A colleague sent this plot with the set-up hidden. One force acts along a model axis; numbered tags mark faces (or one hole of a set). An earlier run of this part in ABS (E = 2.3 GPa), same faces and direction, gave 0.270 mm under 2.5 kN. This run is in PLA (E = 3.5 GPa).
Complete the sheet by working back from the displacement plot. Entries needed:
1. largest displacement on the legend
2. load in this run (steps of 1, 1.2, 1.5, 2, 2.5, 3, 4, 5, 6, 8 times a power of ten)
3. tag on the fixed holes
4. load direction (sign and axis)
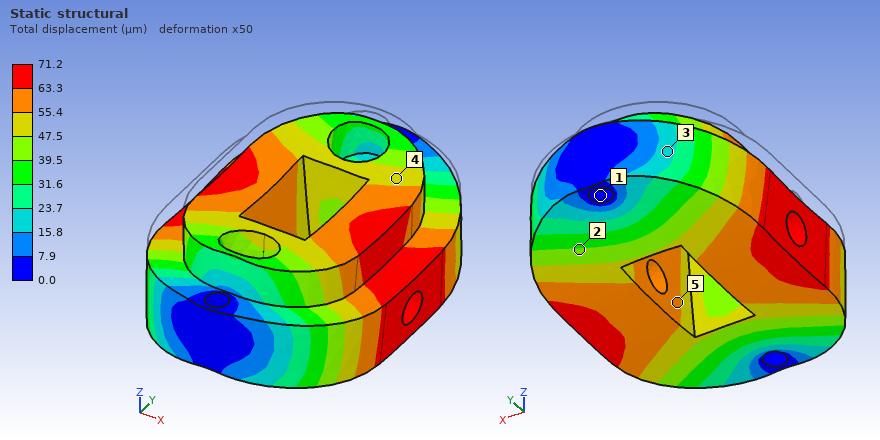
71.2 µm
1 kN
1
-Z
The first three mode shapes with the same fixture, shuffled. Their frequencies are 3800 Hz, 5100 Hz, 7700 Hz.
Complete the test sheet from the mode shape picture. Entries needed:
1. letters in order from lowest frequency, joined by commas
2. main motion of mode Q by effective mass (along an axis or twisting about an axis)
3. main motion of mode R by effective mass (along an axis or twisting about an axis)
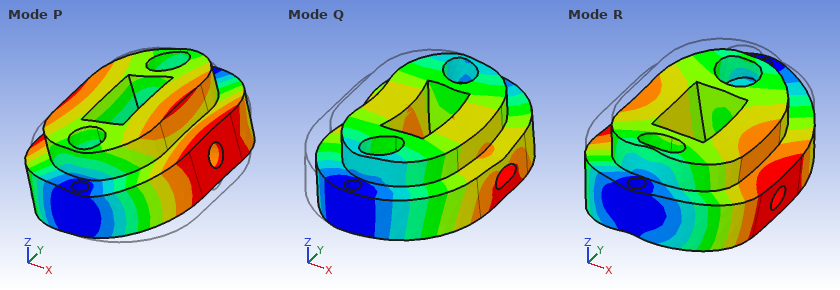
P, R, Q
along X
along Z
